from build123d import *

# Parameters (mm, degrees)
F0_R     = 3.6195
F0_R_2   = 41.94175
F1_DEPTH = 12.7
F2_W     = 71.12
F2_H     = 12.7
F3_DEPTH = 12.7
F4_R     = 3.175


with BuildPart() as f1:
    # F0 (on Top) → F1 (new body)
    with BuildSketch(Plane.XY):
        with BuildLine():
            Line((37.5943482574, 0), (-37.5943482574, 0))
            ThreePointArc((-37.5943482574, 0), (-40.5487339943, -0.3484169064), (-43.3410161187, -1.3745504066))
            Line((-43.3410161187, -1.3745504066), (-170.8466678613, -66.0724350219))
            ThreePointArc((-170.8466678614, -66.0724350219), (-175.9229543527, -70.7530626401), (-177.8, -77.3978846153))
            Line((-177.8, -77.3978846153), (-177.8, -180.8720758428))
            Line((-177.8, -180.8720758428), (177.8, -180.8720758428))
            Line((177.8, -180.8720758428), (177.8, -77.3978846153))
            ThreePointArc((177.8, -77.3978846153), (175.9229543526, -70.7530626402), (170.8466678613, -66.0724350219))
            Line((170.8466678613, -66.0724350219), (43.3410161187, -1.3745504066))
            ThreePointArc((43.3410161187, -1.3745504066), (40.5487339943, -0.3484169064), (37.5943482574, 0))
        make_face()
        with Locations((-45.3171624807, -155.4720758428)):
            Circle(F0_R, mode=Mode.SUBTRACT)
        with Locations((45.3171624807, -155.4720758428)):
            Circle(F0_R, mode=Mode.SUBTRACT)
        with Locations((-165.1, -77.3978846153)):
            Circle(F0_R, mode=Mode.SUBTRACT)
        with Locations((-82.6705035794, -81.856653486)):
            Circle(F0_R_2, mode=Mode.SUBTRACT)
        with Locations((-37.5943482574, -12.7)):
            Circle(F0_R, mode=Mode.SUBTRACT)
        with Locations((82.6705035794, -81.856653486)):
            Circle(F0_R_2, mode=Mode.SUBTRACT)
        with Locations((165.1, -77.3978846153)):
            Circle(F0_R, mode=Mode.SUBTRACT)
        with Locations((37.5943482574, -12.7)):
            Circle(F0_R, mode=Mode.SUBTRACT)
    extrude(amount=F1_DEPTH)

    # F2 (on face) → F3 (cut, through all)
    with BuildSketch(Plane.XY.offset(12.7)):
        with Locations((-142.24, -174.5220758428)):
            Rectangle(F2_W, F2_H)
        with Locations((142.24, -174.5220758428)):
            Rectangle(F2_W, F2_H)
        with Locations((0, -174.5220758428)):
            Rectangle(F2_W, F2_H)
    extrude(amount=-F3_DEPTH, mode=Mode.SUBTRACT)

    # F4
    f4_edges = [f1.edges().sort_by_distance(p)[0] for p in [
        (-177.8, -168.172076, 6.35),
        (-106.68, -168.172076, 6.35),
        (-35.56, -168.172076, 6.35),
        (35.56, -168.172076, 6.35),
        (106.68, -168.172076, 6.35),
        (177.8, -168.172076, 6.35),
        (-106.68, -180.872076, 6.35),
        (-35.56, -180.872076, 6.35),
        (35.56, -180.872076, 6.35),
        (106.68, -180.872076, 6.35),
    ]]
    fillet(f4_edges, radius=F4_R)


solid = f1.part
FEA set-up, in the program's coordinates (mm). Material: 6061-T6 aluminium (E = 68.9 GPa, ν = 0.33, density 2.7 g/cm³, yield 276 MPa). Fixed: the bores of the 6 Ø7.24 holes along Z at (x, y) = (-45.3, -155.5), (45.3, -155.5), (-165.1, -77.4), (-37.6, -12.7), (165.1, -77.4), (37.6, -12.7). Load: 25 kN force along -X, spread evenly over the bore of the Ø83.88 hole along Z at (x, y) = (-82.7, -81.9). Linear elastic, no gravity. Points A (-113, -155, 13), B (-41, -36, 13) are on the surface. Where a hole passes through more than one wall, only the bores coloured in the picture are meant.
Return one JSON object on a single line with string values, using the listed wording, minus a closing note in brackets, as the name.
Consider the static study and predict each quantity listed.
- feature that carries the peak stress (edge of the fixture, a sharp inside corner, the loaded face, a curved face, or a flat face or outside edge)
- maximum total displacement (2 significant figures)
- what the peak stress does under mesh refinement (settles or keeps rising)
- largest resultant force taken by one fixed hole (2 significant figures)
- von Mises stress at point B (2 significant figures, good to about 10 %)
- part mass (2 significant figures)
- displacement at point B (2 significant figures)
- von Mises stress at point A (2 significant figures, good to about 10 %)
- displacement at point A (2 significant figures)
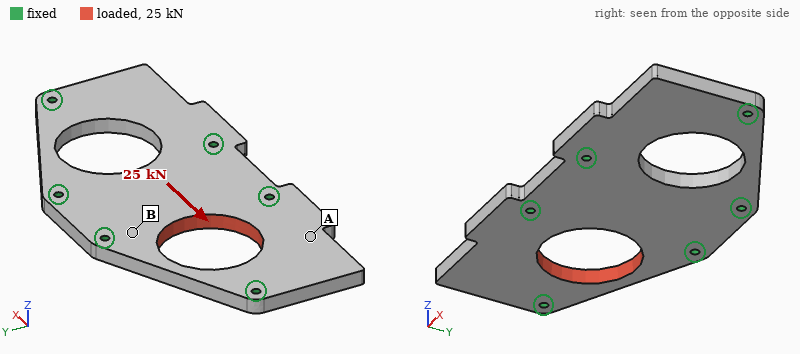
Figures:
{"feature that carries the peak stress": "edge of the fixture", "maximum total displacement": "27 µm", "what the peak stress does under mesh refinement": "keeps rising", "largest resultant force taken by one fixed hole": "6.7 kN", "von Mises stress at point B": "9.9 MPa", "part mass": "1.4 kg", "displacement at point B": "9.4 µm", "von Mises stress at point A": "4.7 MPa", "displacement at point A": "9.0 µm"}
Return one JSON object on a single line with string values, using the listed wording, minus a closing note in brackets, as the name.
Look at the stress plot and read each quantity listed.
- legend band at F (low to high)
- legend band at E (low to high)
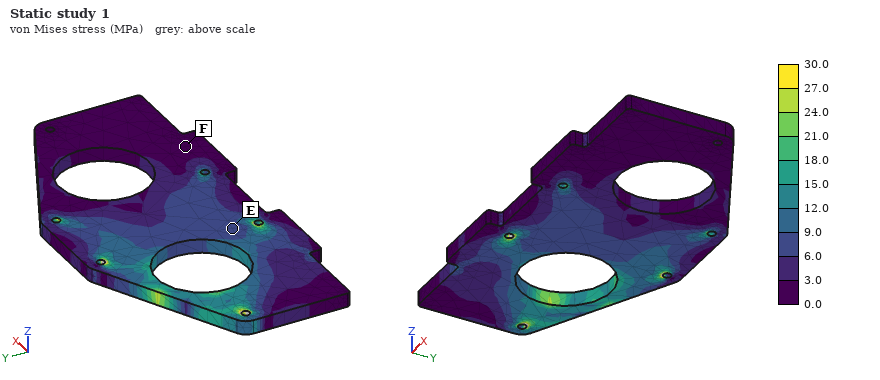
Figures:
{"legend band at F": "0.0 to 3.0 MPa", "legend band at E": "6.0 to 9.0 MPa"}
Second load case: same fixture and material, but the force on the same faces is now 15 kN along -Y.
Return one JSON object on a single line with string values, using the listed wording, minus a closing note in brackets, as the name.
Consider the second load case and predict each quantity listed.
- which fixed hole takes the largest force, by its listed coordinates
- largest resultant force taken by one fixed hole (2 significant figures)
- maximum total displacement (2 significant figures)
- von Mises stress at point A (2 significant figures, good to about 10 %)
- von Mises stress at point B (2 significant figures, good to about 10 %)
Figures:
{"which fixed hole takes the largest force, by its listed coordinates": "(-165.1, -77.4)", "largest resultant force taken by one fixed hole": "5.7 kN", "maximum total displacement": "38 µm", "von Mises stress at point A": "6.1 MPa", "von Mises stress at point B": "10.0 MPa"}
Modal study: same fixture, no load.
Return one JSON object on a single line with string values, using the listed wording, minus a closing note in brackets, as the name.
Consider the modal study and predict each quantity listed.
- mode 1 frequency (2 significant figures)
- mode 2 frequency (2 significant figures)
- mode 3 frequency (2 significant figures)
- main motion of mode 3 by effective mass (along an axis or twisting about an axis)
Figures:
{"mode 1 frequency": "1600 Hz", "mode 2 frequency": "1600 Hz", "mode 3 frequency": "2800 Hz", "main motion of mode 3 by effective mass": "along Z"}
